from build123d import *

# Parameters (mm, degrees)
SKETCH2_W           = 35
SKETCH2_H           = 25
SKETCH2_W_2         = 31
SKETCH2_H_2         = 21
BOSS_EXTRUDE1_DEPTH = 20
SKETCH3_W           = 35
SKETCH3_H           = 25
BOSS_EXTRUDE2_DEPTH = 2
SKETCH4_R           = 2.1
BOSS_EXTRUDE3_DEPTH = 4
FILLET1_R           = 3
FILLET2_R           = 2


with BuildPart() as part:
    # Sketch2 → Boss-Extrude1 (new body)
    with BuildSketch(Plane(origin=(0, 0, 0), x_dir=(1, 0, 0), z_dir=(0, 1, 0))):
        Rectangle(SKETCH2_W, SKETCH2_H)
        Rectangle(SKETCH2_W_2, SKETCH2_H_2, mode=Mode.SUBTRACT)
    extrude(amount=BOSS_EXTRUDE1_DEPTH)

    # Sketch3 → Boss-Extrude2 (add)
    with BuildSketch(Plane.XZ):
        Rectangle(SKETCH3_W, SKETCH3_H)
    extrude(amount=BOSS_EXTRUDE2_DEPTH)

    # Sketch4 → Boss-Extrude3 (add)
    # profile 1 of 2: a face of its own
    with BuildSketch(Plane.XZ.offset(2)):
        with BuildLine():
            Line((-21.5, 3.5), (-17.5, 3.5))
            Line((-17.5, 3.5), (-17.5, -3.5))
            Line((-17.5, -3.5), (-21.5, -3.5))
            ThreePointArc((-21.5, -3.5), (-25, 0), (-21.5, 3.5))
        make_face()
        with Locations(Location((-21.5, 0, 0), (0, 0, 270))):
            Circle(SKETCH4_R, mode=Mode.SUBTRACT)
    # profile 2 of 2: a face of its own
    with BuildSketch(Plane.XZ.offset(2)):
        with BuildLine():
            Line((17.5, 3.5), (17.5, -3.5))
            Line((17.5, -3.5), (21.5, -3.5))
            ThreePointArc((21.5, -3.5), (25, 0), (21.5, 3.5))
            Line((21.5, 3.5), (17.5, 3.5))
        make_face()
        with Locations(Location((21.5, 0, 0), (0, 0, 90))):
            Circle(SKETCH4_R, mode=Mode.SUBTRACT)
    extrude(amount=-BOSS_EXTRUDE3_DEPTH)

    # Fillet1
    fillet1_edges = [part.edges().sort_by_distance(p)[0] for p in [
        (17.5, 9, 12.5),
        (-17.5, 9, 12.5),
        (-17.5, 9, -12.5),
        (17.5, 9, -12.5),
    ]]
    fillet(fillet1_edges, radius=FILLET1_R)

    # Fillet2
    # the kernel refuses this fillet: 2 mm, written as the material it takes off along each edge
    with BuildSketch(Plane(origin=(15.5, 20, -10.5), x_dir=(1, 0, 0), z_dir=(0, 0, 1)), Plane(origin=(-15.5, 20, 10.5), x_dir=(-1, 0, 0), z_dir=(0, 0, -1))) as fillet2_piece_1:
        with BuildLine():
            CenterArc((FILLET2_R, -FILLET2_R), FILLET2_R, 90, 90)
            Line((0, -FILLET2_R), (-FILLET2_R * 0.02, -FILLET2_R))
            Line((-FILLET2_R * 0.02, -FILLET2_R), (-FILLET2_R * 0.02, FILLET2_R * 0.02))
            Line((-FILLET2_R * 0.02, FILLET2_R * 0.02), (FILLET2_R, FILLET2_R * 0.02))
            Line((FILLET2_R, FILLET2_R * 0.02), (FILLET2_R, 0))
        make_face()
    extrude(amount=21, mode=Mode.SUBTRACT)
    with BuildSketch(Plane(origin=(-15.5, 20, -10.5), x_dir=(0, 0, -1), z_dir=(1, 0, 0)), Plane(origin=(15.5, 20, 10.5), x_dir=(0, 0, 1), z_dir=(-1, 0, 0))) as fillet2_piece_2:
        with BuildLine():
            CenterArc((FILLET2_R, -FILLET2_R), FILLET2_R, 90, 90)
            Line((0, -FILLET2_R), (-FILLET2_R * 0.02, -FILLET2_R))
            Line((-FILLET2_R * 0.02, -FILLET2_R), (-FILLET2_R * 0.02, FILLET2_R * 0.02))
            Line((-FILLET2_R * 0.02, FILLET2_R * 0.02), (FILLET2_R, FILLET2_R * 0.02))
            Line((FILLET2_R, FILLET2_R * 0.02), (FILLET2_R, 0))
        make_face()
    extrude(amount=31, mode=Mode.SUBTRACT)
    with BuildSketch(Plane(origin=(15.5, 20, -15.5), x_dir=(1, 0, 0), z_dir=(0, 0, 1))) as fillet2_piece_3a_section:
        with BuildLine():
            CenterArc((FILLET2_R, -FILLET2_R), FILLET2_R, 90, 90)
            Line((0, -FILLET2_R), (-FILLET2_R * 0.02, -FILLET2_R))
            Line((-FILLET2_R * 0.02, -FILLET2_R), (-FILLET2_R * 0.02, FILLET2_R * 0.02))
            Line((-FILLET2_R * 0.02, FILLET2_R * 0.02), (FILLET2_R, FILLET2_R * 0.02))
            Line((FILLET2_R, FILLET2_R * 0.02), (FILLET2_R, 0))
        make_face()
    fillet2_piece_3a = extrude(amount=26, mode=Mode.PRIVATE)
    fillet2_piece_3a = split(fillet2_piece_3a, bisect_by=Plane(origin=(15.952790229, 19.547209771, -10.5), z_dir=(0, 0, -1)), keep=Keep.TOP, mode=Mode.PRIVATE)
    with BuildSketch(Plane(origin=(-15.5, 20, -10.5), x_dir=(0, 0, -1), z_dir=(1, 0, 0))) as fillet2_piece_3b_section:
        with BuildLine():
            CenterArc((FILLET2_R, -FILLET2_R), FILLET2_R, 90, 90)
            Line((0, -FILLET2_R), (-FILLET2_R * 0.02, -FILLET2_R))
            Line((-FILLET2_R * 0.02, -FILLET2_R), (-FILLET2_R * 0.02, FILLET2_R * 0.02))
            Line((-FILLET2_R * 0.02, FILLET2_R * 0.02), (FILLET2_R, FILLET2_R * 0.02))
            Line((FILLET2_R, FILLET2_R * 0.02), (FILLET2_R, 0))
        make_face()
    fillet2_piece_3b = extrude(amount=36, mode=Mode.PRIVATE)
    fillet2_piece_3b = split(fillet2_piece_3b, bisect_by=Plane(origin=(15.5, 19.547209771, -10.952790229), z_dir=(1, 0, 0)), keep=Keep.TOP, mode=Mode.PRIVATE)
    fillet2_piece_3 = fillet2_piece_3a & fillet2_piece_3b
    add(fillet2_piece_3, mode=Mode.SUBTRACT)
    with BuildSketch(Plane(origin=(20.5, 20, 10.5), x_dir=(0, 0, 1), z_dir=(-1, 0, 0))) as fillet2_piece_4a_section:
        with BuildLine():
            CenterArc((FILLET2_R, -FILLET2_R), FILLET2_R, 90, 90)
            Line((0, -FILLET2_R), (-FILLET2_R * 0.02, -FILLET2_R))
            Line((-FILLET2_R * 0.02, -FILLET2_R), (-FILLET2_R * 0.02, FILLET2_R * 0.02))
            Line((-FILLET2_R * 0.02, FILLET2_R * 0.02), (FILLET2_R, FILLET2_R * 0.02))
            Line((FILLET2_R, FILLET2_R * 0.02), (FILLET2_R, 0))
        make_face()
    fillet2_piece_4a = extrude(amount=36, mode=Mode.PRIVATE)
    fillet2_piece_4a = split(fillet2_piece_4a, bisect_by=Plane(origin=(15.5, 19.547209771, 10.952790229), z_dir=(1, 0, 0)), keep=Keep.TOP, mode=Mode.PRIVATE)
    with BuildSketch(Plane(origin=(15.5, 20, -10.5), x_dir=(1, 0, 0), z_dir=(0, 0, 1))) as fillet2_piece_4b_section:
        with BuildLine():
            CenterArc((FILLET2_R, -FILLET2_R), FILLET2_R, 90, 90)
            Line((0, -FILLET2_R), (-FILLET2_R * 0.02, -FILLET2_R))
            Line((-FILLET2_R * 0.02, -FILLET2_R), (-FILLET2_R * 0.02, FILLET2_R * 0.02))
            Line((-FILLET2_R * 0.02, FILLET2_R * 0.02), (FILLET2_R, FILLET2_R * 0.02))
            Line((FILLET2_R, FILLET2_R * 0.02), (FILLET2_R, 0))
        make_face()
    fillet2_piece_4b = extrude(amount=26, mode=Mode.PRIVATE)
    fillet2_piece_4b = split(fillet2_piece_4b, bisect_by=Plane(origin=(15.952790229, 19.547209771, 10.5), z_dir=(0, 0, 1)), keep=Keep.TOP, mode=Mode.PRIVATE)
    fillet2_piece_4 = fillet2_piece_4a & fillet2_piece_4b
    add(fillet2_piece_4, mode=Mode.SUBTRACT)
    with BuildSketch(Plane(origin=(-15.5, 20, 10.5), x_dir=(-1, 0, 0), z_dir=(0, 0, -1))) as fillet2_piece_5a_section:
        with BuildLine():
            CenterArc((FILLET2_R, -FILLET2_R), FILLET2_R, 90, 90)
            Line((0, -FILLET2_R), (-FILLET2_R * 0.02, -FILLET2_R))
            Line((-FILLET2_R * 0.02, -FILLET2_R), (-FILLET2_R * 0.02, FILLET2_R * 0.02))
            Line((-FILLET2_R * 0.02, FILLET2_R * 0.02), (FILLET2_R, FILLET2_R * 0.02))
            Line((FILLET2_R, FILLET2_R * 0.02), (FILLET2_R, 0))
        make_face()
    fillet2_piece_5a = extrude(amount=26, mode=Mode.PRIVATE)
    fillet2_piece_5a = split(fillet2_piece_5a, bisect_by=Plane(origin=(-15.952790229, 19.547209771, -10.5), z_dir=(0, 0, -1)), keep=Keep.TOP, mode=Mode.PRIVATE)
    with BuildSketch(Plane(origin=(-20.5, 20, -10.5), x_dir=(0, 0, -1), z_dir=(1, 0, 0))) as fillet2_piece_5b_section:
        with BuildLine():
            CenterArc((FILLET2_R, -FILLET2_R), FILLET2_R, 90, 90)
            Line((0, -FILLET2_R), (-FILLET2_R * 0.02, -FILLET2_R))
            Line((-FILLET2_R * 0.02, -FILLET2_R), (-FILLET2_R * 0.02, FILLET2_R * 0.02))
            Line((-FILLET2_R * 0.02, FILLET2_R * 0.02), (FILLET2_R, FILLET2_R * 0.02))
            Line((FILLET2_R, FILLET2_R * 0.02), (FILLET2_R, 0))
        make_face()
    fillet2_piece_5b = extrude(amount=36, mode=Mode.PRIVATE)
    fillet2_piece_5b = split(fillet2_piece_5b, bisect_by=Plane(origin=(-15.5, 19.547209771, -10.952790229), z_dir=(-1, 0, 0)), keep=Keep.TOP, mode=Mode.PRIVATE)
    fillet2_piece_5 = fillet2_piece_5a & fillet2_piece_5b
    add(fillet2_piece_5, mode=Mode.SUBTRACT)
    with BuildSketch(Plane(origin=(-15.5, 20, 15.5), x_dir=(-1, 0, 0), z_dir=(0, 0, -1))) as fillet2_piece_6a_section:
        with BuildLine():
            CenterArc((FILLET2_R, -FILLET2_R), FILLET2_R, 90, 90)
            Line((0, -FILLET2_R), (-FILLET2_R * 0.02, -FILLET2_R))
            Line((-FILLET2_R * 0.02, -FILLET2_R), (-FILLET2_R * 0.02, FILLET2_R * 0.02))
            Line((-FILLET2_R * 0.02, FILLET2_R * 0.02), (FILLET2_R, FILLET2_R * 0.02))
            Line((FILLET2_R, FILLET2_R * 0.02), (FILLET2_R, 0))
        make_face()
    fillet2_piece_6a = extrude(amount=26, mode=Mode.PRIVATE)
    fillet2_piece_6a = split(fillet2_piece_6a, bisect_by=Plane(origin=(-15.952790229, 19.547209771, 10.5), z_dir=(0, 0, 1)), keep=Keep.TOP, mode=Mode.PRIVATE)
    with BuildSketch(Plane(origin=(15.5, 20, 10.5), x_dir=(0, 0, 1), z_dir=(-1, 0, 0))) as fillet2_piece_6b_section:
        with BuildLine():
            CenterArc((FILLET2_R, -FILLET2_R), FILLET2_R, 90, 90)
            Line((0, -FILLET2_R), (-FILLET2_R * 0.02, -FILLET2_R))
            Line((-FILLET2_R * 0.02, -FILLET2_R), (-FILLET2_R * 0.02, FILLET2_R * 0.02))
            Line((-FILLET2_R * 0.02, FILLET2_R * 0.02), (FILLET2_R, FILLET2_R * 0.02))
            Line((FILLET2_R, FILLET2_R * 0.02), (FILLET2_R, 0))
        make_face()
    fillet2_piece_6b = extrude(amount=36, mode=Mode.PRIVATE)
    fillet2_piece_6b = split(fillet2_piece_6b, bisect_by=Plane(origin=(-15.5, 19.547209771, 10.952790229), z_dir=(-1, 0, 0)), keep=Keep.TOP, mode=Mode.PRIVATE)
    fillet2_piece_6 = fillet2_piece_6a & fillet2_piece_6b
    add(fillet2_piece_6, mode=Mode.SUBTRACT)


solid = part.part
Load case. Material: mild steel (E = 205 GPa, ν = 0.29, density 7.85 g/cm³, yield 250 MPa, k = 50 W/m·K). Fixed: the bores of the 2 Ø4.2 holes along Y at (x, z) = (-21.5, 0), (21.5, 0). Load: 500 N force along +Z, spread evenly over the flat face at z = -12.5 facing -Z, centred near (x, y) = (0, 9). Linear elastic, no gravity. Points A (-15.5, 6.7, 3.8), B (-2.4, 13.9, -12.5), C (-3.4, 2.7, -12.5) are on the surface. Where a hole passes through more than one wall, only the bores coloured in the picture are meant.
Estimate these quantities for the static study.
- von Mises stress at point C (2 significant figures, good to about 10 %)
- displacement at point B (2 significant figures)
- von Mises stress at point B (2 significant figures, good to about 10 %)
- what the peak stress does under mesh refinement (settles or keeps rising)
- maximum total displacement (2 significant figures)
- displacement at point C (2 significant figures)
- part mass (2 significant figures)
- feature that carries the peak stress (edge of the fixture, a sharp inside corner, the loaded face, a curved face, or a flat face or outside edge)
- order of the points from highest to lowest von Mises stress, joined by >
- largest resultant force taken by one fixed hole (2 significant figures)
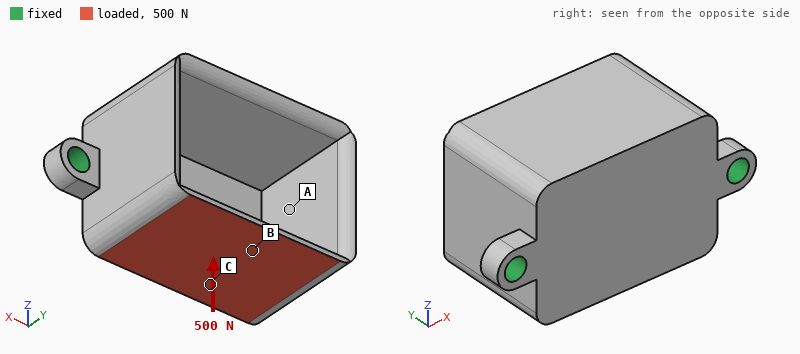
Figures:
25 MPa
39 µm
44 MPa
keeps rising
55 µm
17 µm
49 g
edge of the fixture
B > C > A
260 N
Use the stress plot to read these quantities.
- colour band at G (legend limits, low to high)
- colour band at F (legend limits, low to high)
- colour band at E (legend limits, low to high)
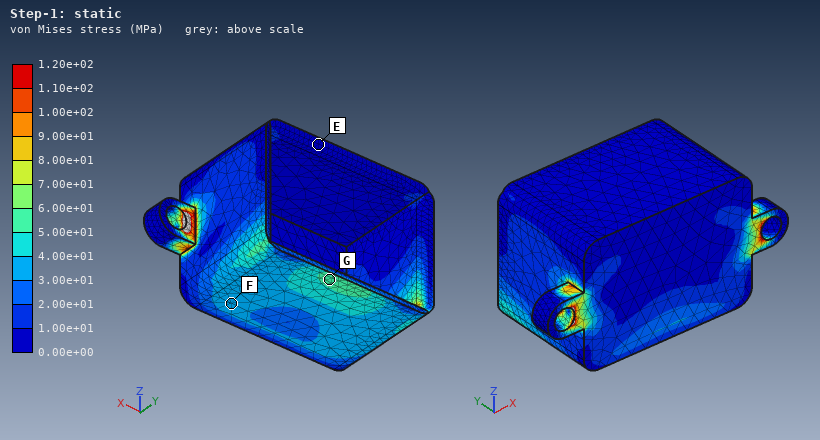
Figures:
5.00e+01 to 6.00e+01 MPa
3.00e+01 to 4.00e+01 MPa
0.00e+00 to 1.00e+01 MPa
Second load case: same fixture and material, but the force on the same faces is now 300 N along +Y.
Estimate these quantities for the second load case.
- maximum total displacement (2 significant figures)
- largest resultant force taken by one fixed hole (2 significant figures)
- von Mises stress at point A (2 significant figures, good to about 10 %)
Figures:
24 µm
150 N
7.7 MPa
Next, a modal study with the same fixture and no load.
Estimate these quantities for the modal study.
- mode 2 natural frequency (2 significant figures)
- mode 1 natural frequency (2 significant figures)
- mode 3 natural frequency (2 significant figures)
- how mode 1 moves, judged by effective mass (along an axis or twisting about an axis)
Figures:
6200 Hz
3700 Hz
8000 Hz
along Z
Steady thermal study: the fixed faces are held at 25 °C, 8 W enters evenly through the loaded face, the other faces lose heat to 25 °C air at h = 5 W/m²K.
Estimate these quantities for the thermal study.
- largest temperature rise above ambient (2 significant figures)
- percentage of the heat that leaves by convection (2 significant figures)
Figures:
39 K
6.4 %
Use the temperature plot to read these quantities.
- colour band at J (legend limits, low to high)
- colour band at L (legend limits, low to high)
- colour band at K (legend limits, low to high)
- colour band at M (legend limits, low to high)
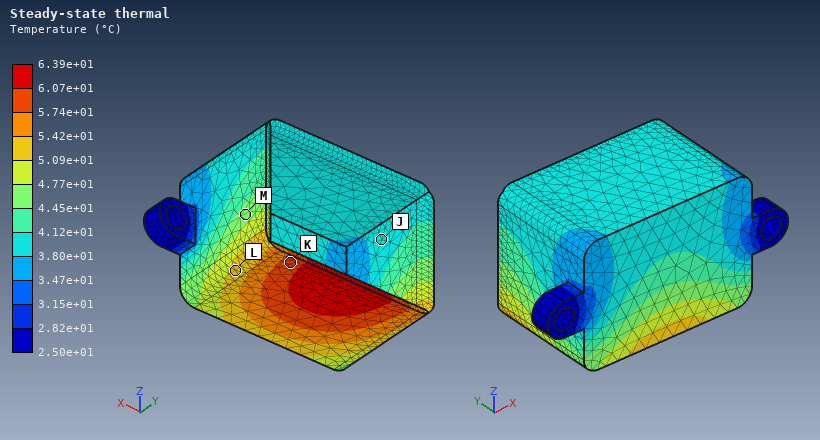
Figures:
3.80e+01 to 4.12e+01 °C
5.09e+01 to 5.42e+01 °C
5.74e+01 to 6.07e+01 °C
4.45e+01 to 4.77e+01 °C
